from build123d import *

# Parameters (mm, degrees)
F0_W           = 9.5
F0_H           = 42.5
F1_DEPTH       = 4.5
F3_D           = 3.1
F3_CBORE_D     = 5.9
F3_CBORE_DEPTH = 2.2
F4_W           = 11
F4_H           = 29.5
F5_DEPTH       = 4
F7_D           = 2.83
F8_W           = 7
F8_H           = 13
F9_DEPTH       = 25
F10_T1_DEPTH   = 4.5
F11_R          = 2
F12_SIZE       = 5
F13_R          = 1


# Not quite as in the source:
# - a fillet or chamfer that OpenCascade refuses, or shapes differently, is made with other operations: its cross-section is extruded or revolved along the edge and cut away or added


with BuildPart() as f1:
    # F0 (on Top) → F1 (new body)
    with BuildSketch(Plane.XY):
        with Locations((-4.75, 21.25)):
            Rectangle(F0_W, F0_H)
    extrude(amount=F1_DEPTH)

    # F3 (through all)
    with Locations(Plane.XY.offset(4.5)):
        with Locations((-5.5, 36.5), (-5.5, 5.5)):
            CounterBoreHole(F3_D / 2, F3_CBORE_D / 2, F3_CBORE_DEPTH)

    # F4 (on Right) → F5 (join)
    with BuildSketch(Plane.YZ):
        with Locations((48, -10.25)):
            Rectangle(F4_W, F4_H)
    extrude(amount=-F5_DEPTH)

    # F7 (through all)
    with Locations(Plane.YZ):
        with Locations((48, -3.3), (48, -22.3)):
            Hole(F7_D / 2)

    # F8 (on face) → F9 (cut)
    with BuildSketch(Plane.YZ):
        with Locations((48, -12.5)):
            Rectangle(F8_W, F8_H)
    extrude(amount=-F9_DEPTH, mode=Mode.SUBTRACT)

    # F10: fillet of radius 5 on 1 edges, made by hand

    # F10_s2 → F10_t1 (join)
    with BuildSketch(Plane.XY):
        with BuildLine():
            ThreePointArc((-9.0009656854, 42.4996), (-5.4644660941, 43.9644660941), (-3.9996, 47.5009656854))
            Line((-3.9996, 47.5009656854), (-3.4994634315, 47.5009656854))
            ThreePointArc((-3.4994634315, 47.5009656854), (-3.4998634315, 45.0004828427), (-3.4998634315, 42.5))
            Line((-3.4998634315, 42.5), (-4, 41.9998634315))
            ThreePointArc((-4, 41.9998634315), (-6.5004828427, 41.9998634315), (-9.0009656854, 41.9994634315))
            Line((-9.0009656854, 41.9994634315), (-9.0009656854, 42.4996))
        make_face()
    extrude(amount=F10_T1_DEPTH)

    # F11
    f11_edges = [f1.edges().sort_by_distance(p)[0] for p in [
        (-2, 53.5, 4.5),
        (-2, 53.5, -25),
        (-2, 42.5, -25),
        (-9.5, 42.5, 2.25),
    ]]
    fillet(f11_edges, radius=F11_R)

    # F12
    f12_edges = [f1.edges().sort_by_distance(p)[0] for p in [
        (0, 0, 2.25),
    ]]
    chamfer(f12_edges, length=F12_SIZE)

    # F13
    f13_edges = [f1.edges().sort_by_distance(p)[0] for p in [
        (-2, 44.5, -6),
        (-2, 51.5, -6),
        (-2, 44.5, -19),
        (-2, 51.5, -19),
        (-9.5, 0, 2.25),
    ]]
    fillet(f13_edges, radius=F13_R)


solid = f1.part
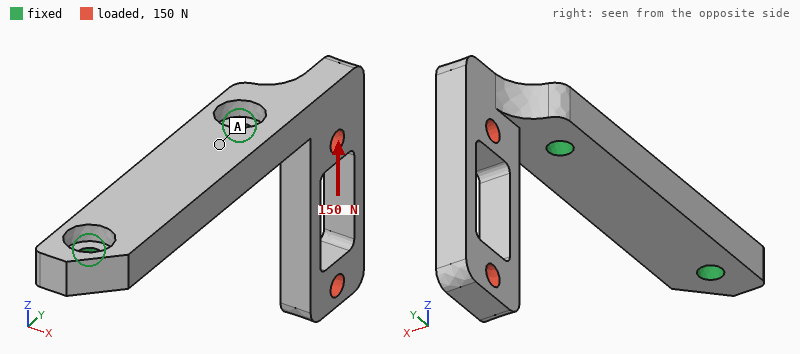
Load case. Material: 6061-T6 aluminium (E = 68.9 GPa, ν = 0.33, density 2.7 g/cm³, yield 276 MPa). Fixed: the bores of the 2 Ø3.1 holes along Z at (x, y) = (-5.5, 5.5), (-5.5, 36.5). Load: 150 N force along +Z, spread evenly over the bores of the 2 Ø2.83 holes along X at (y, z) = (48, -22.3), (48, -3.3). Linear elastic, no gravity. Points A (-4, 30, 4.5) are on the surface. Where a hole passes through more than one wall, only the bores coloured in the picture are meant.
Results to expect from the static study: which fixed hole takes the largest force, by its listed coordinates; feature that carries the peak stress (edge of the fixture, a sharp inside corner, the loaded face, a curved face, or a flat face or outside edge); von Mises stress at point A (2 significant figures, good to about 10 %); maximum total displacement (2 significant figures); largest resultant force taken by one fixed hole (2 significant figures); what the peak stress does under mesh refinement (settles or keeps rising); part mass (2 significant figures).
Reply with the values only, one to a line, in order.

(-5.5, 36.5)
edge of the fixture
12 MPa
0.13 mm
190 N
keeps rising
6.8 g
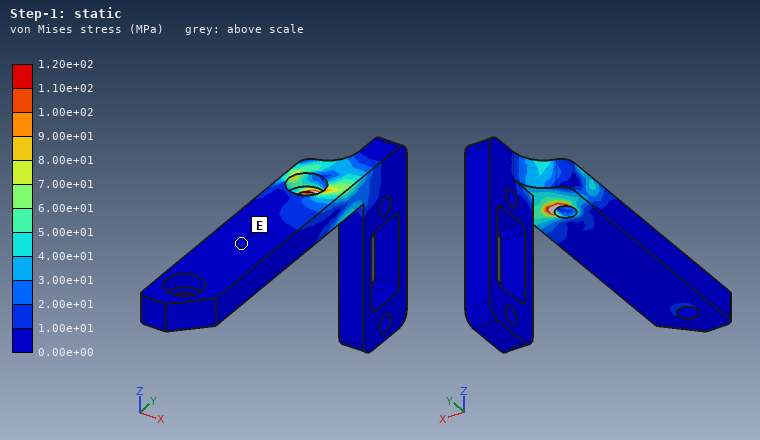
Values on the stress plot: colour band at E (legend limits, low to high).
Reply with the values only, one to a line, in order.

0.00e+00 to 1.00e+01 MPa
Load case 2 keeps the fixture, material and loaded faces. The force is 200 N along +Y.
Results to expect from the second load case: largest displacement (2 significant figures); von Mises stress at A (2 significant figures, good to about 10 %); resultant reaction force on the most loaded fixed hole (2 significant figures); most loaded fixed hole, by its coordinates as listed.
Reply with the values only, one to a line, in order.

0.39 mm
18 MPa
320 N
(-5.5, 36.5)
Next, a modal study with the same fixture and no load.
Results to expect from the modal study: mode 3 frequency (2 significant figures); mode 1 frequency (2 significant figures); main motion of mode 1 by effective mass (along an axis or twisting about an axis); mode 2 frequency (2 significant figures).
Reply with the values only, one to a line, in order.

9600 Hz
2800 Hz
along X
3000 Hz
